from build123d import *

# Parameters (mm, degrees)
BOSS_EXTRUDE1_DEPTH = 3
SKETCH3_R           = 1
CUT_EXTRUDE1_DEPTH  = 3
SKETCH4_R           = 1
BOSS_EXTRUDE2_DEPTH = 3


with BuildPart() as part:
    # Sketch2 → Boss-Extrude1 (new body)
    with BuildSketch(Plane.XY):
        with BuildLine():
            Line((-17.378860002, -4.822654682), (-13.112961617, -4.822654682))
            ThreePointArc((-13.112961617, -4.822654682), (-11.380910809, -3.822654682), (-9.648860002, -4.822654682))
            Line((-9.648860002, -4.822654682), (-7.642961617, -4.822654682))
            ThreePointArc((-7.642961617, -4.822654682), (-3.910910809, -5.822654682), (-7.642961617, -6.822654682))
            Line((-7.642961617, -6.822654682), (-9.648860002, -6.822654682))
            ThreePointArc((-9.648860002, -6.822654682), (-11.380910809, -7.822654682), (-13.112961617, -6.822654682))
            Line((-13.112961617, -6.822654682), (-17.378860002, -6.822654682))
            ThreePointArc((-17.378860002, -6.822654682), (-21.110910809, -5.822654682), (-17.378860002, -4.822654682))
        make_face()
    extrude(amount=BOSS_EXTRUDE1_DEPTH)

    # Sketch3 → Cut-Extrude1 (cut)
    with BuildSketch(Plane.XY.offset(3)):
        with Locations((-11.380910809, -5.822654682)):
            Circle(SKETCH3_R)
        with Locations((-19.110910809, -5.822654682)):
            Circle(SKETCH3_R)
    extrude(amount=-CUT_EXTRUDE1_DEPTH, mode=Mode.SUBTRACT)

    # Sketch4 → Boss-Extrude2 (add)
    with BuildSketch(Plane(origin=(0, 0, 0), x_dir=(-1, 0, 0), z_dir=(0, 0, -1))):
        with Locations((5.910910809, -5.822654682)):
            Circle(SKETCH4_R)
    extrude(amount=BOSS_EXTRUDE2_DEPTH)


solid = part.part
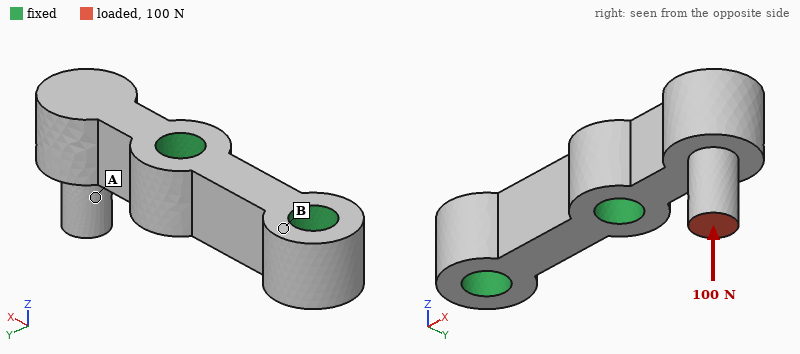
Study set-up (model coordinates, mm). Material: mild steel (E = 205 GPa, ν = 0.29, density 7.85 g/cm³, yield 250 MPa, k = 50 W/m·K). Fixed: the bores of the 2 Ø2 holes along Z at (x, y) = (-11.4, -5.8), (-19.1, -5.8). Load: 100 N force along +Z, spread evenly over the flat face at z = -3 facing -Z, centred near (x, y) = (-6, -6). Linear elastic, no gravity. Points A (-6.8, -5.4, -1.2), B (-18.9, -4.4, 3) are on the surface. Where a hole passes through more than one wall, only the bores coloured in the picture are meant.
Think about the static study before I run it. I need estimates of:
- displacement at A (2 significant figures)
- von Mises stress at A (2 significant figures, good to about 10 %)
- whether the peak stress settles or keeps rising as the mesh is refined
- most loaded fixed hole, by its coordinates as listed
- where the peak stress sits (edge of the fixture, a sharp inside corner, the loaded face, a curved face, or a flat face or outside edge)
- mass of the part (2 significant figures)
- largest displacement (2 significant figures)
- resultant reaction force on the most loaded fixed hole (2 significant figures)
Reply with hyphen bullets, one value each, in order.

- 4.5 µm
- 32 MPa
- keeps rising
- (-11.4, -5.8)
- edge of the fixture
- 1.1 g
- 7.7 µm
- 100 N
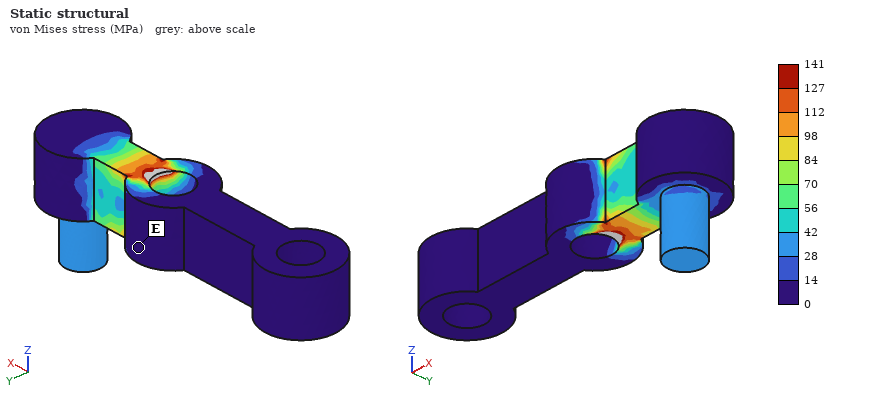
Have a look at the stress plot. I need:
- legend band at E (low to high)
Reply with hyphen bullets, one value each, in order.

- 0 to 14 MPa
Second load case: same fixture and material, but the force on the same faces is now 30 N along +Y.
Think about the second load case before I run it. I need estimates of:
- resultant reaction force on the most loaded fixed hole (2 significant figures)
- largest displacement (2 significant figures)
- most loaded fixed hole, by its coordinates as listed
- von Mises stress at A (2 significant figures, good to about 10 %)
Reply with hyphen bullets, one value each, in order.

- 31 N
- 10 µm
- (-11.4, -5.8)
- 31 MPa
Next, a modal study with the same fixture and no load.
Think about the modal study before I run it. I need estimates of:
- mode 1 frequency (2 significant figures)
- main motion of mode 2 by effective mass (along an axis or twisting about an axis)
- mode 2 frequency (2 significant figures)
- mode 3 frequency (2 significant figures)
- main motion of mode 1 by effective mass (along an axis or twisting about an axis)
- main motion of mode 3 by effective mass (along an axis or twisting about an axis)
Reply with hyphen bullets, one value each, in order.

- 27 kHz
- along Z
- 36 kHz
- 51 kHz
- along Y
- twisting about X
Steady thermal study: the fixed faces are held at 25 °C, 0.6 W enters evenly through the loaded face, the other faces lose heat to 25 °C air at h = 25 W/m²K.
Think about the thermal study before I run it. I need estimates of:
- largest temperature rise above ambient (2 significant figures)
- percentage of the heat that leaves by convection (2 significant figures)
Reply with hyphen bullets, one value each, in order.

- 20 K
- 3.0 %
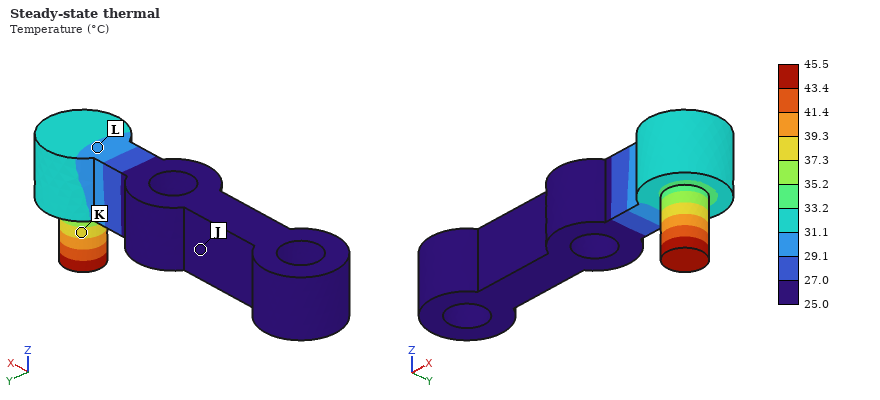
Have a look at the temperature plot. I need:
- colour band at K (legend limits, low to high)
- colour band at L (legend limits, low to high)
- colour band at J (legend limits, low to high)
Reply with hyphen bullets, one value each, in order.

- 37.3 to 39.3 °C
- 29.1 to 31.1 °C
- 25.0 to 27.0 °C
